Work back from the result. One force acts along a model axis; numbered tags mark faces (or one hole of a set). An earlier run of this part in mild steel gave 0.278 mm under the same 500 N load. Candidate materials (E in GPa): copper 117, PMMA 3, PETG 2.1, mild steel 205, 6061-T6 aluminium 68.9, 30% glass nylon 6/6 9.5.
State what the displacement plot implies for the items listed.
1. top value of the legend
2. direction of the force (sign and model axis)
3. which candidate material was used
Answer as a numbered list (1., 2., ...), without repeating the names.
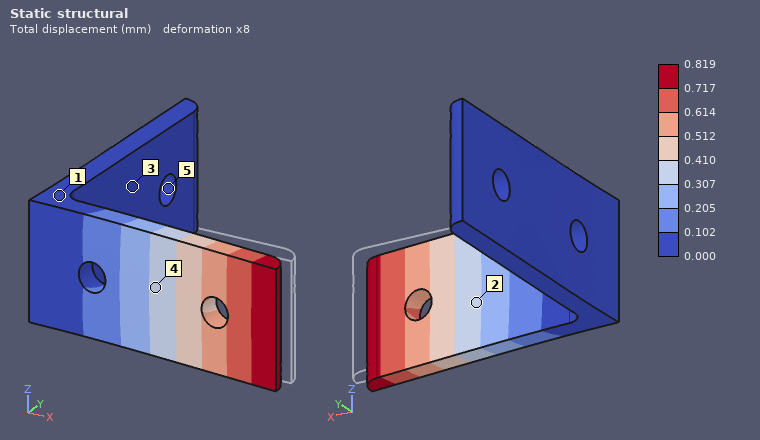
1. 0.819 mm
2. -Y
3. 6061-T6 aluminium
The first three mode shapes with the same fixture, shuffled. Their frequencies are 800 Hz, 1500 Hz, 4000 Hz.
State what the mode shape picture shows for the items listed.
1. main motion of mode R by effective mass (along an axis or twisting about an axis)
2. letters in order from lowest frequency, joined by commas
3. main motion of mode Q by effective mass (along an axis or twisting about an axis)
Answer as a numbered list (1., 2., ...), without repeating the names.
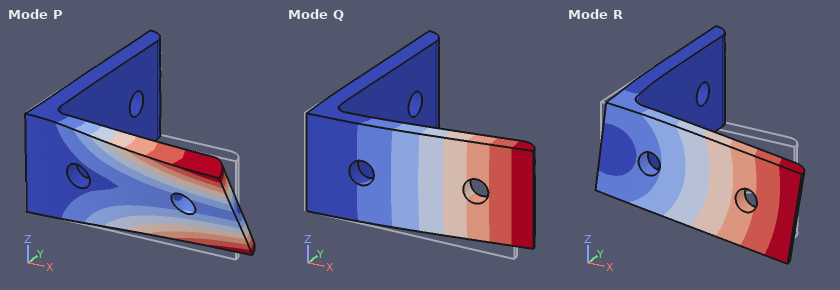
1. along Z
2. Q, R, P
3. along Y
